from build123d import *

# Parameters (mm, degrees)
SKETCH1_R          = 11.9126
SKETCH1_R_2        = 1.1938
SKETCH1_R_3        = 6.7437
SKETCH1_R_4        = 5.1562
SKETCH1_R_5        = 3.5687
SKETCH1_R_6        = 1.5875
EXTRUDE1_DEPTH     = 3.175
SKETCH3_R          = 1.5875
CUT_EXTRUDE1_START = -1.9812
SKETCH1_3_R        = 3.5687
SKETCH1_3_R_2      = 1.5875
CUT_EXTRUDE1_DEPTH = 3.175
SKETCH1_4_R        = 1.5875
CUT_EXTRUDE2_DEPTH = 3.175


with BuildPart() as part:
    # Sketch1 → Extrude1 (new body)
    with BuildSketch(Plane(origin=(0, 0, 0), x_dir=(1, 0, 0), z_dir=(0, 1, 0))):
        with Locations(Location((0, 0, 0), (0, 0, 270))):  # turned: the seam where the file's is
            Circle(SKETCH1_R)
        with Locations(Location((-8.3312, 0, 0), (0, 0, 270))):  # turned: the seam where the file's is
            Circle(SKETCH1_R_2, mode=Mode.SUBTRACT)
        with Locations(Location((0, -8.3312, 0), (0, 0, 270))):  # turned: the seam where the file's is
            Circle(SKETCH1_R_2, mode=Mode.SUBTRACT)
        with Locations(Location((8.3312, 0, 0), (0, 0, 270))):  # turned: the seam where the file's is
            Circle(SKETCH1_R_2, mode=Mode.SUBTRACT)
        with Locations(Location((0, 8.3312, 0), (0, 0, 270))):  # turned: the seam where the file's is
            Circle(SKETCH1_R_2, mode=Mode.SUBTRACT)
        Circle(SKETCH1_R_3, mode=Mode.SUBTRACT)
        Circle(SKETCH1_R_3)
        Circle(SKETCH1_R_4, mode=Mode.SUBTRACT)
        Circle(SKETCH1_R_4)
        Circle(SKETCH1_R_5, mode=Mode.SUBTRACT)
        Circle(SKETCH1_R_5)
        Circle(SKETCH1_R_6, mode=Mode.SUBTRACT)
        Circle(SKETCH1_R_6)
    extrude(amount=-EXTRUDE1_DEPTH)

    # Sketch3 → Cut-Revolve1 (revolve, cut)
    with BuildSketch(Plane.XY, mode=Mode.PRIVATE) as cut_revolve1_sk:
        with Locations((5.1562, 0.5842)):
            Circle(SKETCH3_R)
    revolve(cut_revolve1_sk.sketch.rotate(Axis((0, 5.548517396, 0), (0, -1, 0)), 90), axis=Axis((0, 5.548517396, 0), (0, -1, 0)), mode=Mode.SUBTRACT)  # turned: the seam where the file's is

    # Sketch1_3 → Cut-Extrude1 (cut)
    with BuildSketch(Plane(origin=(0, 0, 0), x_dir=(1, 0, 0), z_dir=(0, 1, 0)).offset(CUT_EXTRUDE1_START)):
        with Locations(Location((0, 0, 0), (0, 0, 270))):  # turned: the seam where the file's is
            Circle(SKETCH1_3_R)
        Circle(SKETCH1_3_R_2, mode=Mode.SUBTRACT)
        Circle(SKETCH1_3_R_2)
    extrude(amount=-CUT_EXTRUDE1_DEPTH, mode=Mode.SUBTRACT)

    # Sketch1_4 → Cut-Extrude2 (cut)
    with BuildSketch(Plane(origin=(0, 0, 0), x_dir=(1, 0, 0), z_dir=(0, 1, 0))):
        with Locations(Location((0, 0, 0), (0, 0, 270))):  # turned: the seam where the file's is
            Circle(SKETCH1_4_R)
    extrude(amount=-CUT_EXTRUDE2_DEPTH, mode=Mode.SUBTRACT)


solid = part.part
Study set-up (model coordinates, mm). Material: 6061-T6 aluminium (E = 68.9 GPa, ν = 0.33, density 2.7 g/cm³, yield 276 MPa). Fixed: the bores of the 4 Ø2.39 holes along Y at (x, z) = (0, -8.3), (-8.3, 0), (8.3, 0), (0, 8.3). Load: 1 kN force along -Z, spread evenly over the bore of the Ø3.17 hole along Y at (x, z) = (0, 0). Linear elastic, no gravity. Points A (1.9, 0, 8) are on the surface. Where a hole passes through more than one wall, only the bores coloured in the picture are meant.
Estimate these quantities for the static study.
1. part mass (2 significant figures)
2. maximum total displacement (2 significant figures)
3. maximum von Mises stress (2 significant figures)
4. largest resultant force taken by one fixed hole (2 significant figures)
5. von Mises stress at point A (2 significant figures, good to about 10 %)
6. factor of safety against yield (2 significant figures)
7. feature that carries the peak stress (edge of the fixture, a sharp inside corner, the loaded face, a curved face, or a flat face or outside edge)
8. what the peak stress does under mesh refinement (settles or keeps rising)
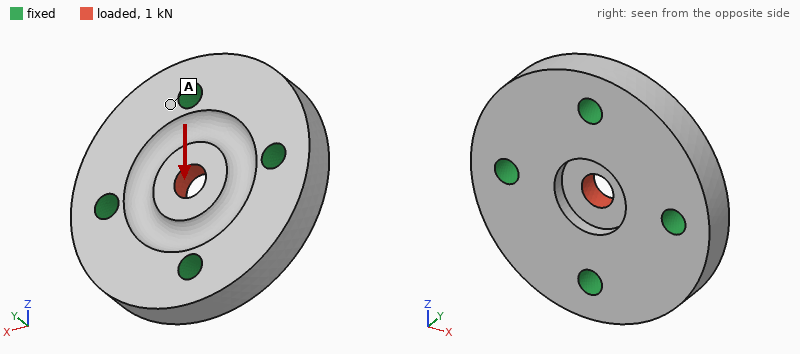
3.3 g
4.7 µm
94 MPa
330 N
9.3 MPa
2.9
the loaded face
settles
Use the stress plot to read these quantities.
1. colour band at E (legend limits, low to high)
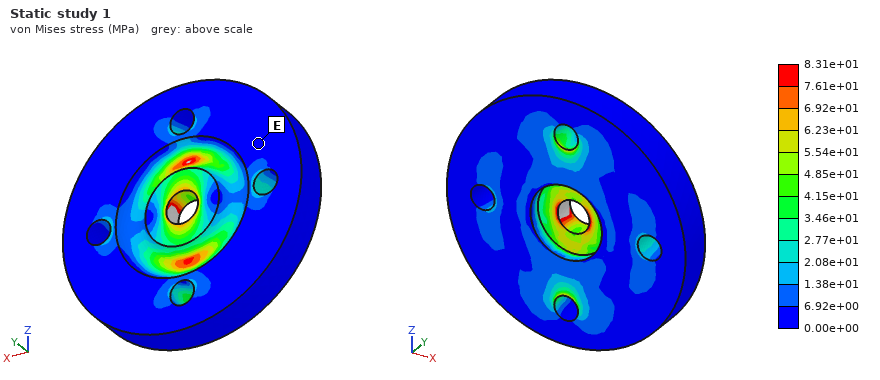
0.00e+00 to 6.92e+00 MPa
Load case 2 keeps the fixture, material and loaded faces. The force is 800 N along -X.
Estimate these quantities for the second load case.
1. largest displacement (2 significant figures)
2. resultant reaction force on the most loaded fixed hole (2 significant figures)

3.7 µm
260 N
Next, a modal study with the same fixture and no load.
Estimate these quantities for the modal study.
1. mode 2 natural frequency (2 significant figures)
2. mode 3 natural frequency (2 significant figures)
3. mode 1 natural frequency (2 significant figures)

62 kHz
62 kHz
60 kHz
